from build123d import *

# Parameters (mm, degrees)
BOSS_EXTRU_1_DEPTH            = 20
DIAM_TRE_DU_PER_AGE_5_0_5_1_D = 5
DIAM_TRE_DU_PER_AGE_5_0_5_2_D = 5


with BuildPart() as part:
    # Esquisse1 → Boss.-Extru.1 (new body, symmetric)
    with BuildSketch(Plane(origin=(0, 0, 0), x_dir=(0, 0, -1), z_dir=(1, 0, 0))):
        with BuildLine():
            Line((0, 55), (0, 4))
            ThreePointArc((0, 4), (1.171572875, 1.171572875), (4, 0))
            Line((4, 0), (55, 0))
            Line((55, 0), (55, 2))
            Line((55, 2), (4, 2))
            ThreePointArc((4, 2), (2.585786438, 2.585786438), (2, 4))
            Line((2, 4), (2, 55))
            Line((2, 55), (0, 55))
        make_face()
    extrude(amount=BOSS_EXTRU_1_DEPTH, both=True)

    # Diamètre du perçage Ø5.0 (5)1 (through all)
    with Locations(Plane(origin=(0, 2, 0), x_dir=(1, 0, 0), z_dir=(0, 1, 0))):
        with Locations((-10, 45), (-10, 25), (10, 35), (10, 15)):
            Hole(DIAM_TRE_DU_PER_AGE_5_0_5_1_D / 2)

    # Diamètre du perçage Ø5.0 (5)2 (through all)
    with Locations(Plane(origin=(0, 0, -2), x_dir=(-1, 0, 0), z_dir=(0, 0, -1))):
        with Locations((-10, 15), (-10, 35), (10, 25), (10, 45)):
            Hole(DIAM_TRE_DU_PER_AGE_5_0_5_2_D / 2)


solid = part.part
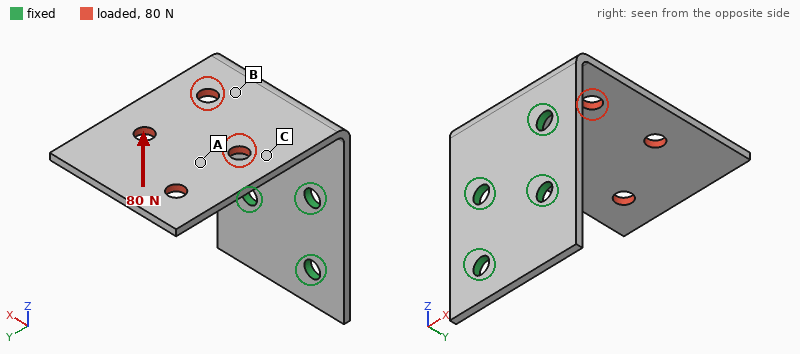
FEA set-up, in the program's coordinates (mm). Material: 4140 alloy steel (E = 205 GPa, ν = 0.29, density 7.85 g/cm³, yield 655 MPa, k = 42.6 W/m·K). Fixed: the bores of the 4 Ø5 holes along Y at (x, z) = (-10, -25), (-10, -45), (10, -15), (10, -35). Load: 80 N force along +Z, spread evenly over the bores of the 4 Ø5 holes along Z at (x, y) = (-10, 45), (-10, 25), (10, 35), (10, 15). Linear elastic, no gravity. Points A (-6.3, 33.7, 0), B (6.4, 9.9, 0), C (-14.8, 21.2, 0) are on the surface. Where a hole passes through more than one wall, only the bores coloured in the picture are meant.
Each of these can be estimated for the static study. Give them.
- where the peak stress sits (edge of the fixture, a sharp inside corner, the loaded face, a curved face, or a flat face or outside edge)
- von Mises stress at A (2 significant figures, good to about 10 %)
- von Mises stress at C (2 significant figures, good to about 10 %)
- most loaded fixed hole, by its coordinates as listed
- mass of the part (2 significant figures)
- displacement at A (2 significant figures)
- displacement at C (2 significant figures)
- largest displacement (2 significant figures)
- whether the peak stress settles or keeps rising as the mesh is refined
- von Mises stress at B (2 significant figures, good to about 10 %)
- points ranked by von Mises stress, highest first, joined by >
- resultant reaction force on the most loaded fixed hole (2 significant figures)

edge of the fixture
12 MPa
34 MPa
(10, -15)
65 g
0.34 mm
0.20 mm
0.62 mm
keeps rising
55 MPa
B > C > A
56 N
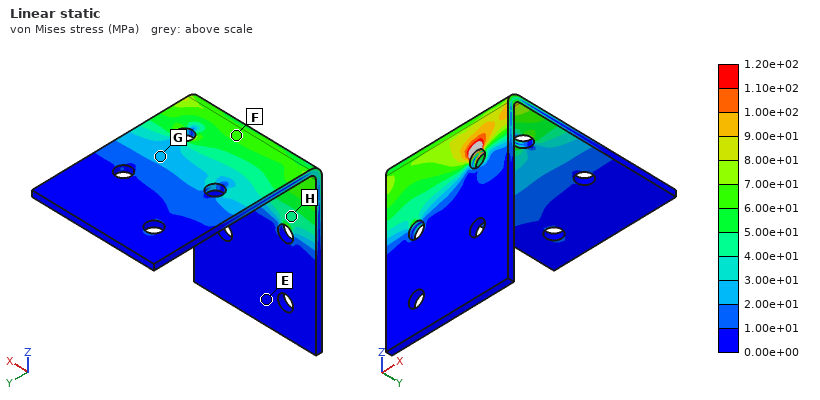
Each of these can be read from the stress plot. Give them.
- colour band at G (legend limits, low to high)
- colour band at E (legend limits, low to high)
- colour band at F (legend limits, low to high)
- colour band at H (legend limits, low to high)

2.00e+01 to 3.00e+01 MPa
0.00e+00 to 1.00e+01 MPa
6.00e+01 to 7.00e+01 MPa
4.00e+01 to 5.00e+01 MPa
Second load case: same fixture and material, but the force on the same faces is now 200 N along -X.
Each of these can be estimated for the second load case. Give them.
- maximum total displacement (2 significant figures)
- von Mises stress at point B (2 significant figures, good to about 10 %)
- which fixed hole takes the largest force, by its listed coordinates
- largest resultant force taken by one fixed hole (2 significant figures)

0.39 mm
32 MPa
(10, -15)
250 N
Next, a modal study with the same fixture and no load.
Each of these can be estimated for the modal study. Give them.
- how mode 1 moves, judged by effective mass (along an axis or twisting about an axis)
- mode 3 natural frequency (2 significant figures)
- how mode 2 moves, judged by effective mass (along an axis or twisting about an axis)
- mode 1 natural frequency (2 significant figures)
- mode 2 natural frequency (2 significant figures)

along Z
1700 Hz
along X
400 Hz
850 Hz
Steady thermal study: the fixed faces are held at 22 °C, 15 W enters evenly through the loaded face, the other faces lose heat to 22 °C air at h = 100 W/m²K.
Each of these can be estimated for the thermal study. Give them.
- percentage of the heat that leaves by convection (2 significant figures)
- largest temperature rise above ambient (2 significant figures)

87 %
42 K
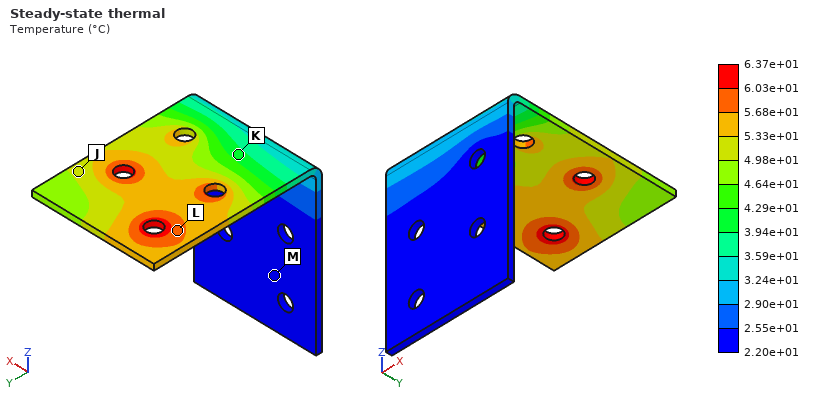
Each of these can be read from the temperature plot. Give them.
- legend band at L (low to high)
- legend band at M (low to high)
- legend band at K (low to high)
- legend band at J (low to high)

5.68e+01 to 6.03e+01 °C
2.20e+01 to 2.55e+01 °C
3.94e+01 to 4.29e+01 °C
4.98e+01 to 5.33e+01 °C
